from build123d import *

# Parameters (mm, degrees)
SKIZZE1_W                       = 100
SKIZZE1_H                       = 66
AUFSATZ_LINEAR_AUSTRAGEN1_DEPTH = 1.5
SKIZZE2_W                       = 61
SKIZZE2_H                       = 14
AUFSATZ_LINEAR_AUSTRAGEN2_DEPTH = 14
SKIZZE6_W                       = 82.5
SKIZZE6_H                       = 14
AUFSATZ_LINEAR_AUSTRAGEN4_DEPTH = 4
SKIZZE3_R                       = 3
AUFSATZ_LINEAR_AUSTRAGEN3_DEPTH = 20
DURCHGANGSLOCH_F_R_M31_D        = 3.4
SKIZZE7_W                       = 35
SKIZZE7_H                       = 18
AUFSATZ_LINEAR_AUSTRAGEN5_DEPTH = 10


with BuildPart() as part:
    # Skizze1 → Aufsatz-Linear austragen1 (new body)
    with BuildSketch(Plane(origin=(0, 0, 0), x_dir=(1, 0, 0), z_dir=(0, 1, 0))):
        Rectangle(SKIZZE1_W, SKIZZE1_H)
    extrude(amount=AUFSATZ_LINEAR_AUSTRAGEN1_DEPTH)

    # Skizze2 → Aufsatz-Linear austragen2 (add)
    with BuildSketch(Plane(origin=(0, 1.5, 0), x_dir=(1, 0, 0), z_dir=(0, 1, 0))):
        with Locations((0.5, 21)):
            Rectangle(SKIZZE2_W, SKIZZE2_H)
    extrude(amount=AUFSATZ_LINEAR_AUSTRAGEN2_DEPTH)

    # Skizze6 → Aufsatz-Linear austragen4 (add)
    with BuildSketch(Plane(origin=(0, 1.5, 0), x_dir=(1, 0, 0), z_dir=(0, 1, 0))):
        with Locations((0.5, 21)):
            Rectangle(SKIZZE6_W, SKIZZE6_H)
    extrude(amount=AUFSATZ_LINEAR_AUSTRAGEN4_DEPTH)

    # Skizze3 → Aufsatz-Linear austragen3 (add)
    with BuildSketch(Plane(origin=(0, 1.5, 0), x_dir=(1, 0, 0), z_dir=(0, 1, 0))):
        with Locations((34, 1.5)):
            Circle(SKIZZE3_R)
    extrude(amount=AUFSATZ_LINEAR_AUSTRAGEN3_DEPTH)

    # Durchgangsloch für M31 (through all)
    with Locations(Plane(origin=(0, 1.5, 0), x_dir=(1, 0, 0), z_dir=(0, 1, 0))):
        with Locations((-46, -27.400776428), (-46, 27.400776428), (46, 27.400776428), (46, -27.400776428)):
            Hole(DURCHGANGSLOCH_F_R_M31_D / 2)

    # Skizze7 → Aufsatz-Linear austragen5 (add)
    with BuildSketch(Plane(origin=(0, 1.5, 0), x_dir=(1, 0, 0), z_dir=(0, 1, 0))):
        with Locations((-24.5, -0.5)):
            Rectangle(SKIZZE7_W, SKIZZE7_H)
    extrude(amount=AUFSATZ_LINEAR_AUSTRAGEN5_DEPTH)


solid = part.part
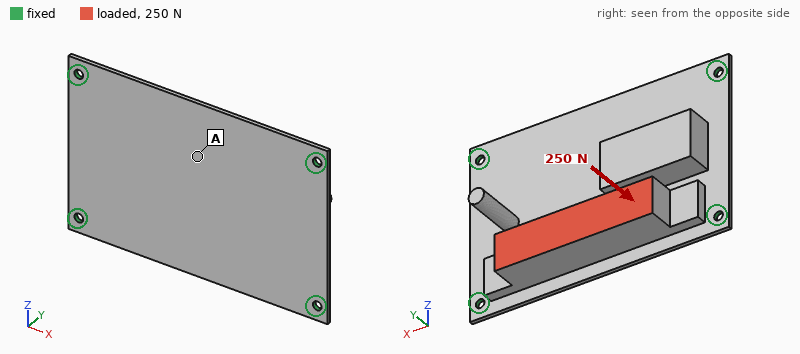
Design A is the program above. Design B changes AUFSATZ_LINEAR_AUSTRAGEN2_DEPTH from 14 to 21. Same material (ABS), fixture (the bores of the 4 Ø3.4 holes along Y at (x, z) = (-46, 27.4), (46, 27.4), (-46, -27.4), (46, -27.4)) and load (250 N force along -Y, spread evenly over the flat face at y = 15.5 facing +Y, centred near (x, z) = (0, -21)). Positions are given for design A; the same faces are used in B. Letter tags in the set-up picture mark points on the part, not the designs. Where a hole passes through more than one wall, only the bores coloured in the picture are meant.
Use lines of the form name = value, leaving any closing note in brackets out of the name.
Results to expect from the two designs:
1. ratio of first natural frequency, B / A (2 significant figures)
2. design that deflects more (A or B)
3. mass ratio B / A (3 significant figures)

ratio of first natural frequency, B / A = 0.88
design that deflects more = B
mass ratio B / A = 1.20
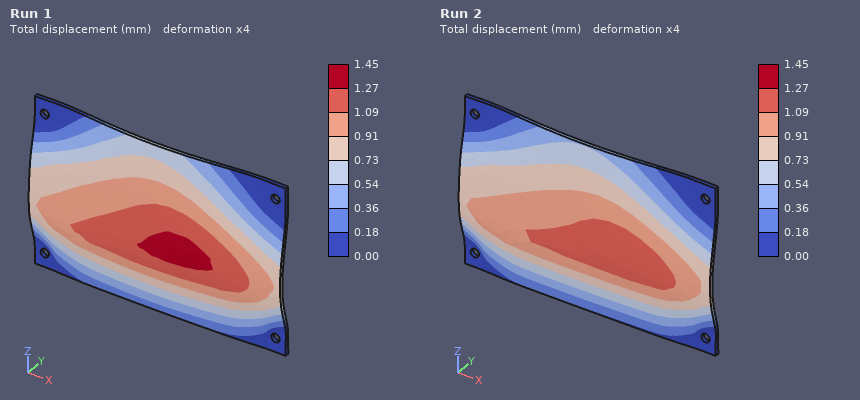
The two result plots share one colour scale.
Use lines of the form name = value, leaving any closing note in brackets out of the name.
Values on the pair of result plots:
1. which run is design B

which run is design B = Run 2
